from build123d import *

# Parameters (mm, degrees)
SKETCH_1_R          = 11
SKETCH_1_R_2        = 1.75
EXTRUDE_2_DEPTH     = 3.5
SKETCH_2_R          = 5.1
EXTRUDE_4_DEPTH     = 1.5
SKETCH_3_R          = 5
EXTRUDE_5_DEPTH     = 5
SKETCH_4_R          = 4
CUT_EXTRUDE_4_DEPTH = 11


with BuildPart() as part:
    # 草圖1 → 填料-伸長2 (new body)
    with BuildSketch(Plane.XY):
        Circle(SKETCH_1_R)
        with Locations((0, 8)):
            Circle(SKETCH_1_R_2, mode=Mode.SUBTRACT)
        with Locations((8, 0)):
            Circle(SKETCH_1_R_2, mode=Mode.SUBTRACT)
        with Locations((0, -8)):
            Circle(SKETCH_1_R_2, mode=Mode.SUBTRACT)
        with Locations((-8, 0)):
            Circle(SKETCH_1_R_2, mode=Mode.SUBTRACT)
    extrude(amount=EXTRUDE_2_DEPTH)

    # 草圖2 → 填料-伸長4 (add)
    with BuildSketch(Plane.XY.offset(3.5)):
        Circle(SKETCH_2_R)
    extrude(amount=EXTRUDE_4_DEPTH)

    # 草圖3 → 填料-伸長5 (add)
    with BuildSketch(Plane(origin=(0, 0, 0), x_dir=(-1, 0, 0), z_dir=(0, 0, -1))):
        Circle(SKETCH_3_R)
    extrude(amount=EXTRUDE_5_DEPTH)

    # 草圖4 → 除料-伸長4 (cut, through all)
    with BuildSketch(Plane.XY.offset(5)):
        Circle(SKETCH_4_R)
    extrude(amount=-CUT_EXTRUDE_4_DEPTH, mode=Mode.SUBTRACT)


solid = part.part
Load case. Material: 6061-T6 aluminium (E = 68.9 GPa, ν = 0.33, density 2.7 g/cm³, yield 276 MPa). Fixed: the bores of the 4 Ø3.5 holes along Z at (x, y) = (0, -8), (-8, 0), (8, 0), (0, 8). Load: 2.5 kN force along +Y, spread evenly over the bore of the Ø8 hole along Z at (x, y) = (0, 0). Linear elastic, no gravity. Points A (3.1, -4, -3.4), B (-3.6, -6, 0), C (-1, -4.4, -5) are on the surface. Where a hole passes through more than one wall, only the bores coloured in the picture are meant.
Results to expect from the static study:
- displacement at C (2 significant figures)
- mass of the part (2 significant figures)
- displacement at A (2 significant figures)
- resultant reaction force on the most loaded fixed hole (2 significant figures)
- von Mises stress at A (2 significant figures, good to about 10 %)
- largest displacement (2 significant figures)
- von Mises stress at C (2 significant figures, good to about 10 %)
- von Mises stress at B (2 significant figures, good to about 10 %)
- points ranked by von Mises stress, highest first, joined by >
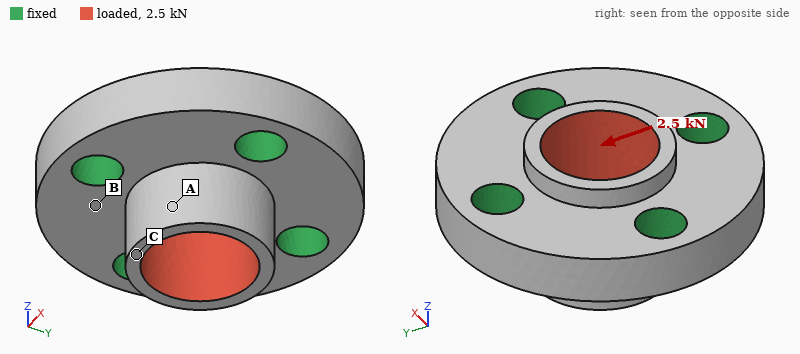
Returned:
17 µm
3.3 g
13 µm
770 N
40 MPa
17 µm
65 MPa
17 MPa
C > A > B
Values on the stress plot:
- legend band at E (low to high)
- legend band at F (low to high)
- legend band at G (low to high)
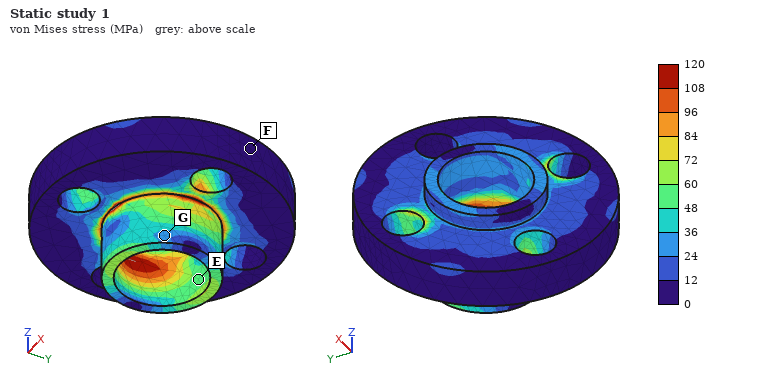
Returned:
48 to 60 MPa
0 to 12 MPa
24 to 36 MPa
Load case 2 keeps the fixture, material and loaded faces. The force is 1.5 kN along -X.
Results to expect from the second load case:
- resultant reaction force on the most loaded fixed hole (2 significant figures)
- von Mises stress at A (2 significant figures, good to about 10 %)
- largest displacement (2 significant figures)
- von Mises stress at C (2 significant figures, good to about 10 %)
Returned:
460 N
25 MPa
10 µm
9.1 MPa
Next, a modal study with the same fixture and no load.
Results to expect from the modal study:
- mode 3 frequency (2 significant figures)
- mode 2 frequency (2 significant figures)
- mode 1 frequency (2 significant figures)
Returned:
82 kHz
71 kHz
67 kHz
